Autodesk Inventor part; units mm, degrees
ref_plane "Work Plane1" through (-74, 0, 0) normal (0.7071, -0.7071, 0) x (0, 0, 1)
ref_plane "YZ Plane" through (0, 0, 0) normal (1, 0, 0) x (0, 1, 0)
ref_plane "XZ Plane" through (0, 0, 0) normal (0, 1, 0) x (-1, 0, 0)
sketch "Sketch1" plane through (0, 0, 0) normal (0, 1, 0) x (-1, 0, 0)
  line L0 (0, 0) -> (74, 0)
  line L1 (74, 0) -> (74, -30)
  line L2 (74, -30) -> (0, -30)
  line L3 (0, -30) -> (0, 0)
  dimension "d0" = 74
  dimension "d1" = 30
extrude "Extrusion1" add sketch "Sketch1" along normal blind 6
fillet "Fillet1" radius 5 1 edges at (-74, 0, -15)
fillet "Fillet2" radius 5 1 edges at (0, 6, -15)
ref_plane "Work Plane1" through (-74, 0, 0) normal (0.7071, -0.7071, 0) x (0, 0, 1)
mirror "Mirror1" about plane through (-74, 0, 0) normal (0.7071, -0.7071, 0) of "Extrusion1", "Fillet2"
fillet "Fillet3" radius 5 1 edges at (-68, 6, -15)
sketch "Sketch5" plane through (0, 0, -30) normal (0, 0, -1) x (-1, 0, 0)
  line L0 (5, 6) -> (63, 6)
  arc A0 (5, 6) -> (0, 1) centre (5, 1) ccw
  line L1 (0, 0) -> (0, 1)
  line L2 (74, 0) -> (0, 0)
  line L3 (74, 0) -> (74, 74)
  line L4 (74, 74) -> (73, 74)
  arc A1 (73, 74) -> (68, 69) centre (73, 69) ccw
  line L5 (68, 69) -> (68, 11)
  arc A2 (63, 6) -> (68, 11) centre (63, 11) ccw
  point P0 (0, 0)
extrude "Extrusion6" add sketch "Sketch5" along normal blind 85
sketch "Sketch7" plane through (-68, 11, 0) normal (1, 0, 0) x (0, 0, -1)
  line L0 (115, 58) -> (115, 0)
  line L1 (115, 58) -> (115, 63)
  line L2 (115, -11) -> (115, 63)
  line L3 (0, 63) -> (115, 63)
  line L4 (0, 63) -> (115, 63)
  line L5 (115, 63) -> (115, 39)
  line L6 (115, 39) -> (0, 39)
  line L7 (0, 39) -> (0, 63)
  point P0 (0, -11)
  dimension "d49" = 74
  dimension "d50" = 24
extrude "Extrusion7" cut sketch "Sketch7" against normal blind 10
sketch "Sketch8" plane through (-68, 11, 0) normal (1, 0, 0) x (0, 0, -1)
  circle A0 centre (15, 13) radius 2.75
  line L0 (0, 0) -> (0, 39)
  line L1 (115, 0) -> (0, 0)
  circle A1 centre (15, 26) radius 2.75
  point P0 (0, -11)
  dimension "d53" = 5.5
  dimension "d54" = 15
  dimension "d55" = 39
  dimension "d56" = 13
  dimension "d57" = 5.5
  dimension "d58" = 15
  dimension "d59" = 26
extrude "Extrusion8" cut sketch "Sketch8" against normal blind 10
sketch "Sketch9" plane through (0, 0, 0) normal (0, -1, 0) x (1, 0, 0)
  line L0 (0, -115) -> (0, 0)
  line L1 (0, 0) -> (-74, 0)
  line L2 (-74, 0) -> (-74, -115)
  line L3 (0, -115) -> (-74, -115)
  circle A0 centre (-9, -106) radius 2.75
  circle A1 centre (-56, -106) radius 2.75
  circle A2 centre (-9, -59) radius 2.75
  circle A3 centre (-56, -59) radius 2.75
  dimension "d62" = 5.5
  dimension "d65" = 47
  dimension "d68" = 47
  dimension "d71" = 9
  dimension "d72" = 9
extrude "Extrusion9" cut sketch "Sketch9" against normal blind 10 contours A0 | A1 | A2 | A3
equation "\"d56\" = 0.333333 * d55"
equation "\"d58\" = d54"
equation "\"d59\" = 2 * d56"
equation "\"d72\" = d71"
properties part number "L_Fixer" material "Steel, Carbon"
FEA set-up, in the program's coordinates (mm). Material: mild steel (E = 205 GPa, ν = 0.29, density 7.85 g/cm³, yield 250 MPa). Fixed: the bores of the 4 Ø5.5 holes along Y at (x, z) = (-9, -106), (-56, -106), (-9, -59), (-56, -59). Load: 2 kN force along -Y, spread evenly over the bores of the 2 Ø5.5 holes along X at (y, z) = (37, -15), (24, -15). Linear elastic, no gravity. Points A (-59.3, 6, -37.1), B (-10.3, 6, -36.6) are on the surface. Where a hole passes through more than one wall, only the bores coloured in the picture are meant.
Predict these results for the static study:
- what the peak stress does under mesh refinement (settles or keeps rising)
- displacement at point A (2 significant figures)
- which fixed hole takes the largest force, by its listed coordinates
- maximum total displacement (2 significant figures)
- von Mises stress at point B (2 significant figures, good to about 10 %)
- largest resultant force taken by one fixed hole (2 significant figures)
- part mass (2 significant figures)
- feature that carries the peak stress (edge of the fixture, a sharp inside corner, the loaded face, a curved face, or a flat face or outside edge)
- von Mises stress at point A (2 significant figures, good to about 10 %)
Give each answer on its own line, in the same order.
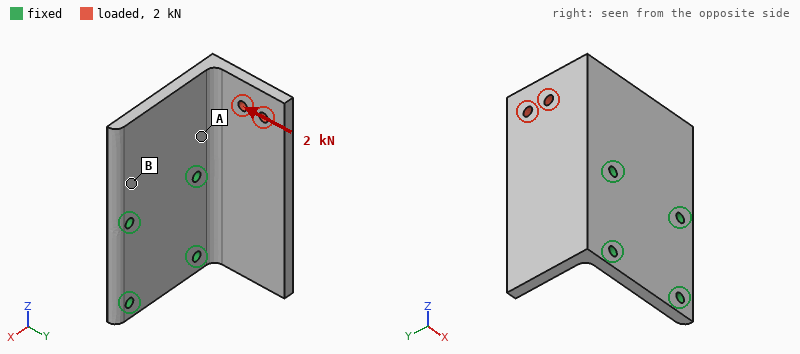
keeps rising
0.024 mm
(-56, -59)
0.12 mm
15 MPa
4.0 kN
630 g
edge of the fixture
34 MPa
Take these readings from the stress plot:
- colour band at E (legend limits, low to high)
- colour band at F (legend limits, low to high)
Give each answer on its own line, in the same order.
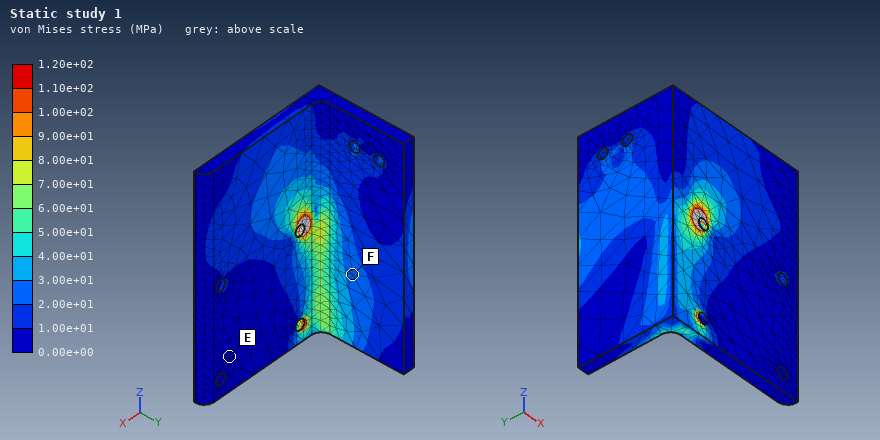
0.00e+00 to 1.00e+01 MPa
2.00e+01 to 3.00e+01 MPa
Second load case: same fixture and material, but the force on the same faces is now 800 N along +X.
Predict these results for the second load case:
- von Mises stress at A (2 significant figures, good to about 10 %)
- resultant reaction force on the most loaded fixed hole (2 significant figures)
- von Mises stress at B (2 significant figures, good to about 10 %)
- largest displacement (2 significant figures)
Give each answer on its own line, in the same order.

37 MPa
780 N
6.7 MPa
0.13 mm
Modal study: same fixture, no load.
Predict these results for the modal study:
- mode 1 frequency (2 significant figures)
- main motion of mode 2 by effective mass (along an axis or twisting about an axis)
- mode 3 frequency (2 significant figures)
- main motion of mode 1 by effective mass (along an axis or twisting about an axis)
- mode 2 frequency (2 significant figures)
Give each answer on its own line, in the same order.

1400 Hz
along Y
2300 Hz
along X
2000 Hz
